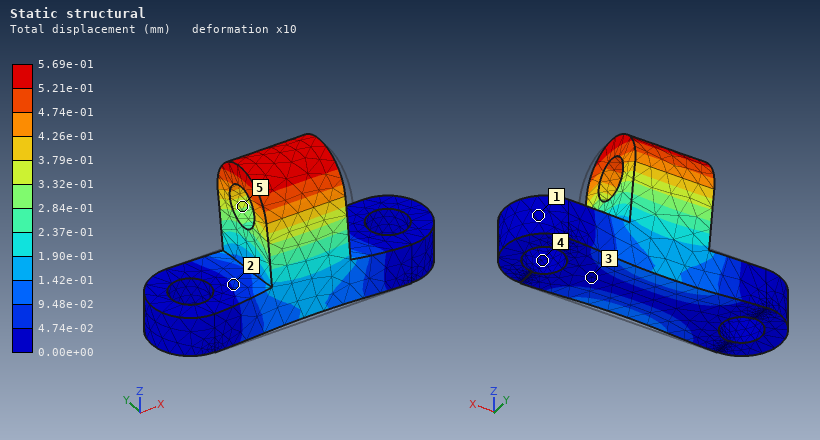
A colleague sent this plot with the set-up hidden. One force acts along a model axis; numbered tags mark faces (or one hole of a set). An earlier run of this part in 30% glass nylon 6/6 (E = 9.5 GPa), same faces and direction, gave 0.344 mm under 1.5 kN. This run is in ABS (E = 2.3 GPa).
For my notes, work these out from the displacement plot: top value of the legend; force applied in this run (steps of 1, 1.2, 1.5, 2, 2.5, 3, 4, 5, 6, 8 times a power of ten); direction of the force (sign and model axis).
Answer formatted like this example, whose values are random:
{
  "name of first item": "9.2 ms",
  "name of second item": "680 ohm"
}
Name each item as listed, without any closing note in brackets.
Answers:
{
  "top value of the legend": "5.69e-01 mm",
  "force applied in this run": "600 N",
  "direction of the force": "+Y"
}
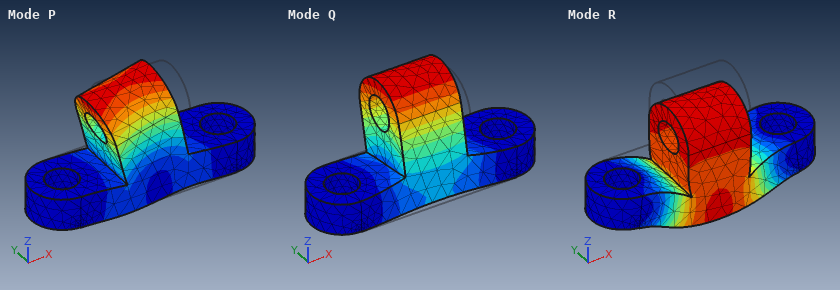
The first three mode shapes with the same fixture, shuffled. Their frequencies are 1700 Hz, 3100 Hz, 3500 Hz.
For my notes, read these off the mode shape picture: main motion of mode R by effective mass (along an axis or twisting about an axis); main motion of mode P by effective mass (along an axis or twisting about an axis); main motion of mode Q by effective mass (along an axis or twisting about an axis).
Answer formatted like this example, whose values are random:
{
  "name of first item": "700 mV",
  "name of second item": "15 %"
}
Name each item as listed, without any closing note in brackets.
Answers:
{
  "main motion of mode R by effective mass": "along Z",
  "main motion of mode P by effective mass": "along X",
  "main motion of mode Q by effective mass": "along Y"
}
